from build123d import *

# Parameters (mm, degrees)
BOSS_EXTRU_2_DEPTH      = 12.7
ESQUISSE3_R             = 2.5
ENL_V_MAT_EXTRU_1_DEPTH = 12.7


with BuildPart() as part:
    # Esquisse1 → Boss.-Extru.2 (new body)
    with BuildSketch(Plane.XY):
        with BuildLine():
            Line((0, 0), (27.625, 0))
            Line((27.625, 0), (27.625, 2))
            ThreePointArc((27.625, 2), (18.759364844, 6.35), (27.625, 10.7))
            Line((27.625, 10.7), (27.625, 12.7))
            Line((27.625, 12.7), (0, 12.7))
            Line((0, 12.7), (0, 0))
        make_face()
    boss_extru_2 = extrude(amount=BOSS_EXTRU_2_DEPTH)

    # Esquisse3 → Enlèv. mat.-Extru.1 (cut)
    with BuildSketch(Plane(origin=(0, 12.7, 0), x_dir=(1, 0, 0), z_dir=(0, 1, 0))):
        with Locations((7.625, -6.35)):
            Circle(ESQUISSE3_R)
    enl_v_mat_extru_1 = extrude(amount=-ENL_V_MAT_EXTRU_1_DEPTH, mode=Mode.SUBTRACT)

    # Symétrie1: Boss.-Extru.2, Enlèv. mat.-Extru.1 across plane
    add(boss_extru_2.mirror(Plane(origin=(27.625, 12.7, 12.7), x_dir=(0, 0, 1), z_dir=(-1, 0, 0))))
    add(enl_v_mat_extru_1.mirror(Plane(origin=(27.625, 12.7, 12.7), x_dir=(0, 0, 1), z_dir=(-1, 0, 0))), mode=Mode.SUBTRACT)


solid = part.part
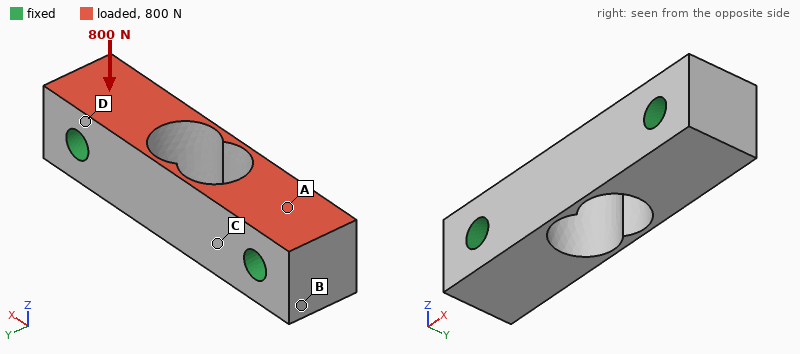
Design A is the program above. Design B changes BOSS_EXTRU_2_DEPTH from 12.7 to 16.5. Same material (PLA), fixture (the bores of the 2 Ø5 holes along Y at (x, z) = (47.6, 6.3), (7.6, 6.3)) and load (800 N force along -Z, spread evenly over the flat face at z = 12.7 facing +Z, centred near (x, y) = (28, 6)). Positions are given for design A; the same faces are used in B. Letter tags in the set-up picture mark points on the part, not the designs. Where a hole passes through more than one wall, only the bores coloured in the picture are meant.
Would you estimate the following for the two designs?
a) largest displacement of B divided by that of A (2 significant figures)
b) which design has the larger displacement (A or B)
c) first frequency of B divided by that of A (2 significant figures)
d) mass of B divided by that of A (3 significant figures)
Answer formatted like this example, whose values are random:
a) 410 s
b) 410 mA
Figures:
a) 0.80
b) A
c) 0.94
d) 1.32
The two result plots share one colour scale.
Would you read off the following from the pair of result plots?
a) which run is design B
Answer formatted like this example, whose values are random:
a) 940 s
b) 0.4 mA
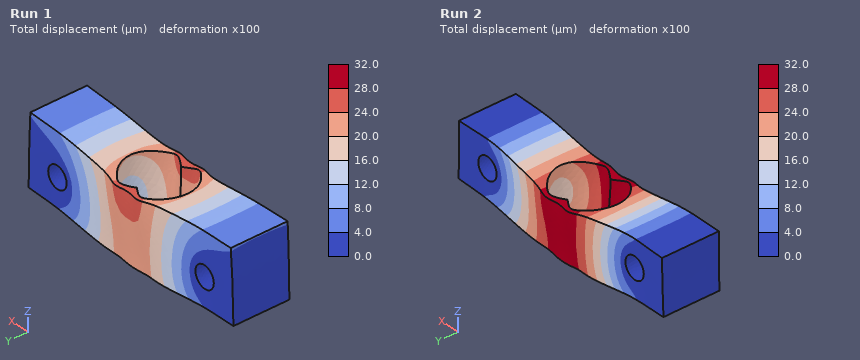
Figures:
a) Run 1
